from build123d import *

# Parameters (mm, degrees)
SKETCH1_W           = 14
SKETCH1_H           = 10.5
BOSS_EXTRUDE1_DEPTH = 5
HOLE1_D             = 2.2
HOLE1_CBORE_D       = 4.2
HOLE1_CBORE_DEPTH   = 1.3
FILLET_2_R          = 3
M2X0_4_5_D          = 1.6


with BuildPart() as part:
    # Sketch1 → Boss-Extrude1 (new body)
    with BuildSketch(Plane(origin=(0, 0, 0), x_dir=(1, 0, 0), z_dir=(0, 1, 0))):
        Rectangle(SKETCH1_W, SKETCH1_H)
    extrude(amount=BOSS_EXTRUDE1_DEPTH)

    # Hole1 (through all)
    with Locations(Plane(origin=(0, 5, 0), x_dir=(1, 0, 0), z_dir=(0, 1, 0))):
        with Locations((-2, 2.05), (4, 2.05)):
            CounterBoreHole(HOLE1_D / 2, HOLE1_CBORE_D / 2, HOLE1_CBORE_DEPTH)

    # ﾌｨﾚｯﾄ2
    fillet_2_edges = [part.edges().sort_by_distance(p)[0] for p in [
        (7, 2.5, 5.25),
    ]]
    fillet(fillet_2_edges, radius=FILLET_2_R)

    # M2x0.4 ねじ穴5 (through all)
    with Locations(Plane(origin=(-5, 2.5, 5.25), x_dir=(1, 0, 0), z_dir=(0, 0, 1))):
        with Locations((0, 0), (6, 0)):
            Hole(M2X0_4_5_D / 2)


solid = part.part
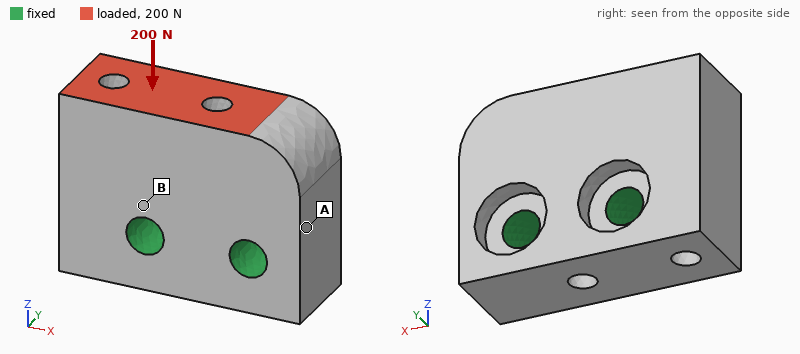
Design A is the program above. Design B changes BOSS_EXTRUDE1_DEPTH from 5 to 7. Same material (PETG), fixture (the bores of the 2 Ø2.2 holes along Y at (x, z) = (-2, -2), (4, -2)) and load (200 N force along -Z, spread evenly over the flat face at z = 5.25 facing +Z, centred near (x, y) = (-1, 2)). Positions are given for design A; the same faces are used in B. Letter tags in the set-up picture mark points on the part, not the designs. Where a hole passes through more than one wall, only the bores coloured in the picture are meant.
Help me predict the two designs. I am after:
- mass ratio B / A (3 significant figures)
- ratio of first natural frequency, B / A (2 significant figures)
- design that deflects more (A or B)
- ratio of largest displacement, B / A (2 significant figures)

1.38
0.81
B
1.5
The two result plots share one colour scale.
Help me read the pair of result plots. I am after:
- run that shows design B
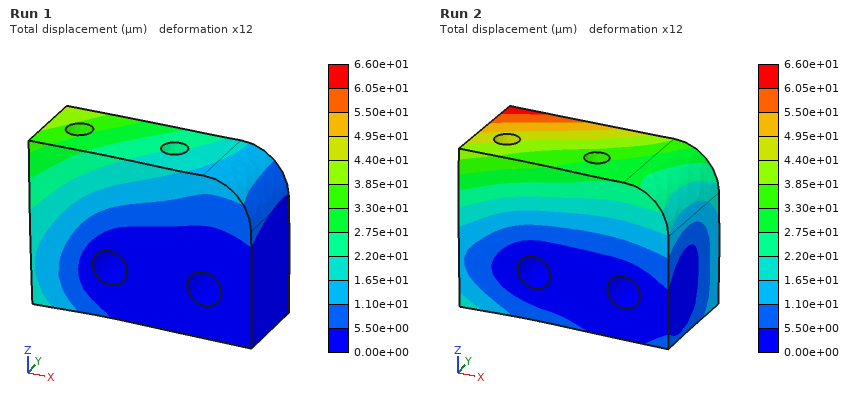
Run 2
